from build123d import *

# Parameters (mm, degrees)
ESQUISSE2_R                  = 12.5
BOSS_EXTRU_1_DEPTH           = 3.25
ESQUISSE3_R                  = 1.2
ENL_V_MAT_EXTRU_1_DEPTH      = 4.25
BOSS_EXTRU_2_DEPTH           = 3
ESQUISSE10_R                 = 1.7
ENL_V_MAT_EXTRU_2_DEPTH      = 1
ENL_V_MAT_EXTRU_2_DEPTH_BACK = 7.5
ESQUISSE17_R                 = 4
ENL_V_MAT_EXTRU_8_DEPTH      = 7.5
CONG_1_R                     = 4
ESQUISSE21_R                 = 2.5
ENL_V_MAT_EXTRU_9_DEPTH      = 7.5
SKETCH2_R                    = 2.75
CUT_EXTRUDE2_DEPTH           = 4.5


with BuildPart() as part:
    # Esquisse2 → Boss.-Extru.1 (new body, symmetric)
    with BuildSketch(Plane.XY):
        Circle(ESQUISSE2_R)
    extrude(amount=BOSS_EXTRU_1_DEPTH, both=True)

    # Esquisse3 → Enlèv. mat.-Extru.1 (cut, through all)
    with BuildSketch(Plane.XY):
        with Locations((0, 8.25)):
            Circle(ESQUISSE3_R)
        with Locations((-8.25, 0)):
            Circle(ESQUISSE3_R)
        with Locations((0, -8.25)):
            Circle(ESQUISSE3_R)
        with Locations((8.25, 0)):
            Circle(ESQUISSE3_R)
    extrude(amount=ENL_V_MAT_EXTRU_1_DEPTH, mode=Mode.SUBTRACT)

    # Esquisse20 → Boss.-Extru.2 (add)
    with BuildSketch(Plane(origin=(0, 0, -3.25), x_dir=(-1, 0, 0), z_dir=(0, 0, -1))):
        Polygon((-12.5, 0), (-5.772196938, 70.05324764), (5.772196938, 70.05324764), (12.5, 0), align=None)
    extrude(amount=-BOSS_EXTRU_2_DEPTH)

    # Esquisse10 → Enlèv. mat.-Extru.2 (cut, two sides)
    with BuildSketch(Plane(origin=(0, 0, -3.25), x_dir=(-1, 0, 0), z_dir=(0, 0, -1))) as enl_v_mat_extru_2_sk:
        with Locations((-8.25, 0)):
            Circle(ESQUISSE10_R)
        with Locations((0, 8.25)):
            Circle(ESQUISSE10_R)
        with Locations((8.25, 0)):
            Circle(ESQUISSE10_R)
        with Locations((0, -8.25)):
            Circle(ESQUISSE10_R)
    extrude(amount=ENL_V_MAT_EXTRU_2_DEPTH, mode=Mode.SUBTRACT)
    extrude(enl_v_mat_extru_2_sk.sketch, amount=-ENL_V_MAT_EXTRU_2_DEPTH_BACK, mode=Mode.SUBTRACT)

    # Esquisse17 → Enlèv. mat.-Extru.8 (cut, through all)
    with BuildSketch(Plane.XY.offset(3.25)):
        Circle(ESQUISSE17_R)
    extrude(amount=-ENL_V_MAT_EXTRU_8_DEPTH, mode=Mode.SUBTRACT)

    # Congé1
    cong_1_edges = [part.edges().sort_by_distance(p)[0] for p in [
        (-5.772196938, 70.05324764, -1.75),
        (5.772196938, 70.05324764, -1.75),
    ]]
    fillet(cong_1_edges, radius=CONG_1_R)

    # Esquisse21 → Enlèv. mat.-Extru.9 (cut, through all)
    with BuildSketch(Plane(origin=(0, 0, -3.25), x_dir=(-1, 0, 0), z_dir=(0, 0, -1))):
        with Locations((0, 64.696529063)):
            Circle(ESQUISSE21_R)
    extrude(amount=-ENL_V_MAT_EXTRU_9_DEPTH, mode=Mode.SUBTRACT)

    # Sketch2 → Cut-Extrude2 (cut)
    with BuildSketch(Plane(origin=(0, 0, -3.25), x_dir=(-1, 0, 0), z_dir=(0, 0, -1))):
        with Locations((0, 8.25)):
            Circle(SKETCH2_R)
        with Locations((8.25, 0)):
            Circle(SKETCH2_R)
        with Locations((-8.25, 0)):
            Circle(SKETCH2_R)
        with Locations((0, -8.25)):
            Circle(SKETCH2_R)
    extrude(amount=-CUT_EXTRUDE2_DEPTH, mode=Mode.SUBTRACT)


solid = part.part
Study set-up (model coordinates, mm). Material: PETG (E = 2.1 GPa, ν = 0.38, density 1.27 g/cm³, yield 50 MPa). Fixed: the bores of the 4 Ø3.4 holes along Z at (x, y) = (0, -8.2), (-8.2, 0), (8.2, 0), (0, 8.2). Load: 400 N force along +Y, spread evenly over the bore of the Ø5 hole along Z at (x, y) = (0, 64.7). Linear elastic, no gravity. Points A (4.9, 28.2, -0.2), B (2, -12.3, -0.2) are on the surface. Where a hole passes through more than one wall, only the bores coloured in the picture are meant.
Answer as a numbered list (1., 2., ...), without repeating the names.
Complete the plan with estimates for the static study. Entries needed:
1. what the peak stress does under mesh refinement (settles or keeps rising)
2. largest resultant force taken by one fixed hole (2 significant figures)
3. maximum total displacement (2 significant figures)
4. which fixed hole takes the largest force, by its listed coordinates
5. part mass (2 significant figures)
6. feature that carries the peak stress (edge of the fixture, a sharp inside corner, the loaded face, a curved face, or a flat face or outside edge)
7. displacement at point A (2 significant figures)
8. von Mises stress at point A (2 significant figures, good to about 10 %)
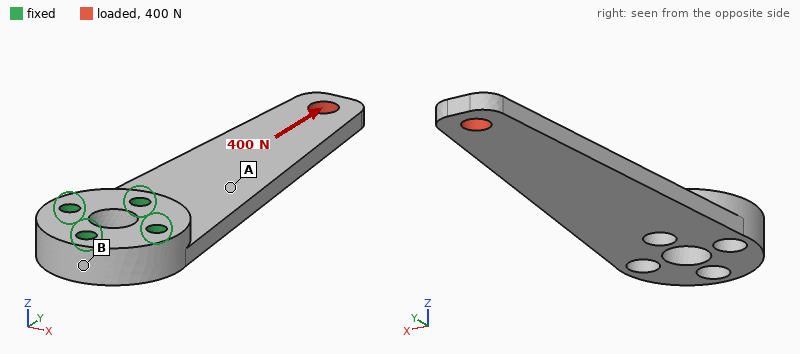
1. keeps rising
2. 150 N
3. 0.62 mm
4. (0, 8.2)
5. 6.8 g
6. edge of the fixture
7. 0.20 mm
8. 6.9 MPa
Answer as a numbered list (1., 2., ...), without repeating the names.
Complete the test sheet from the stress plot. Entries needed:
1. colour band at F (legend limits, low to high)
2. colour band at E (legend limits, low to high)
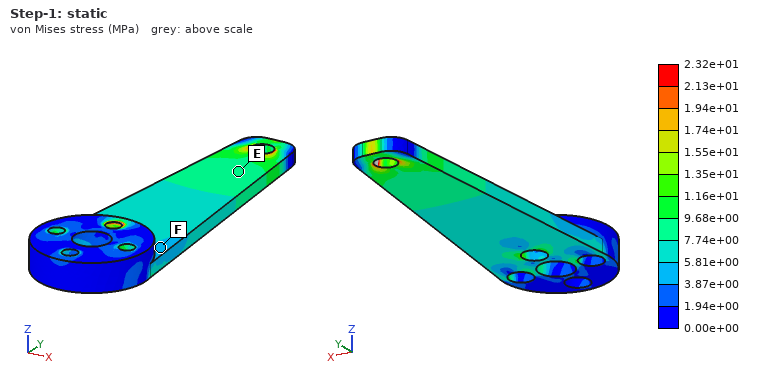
1. 3.87e+00 to 5.81e+00 MPa
2. 7.74e+00 to 9.68e+00 MPa
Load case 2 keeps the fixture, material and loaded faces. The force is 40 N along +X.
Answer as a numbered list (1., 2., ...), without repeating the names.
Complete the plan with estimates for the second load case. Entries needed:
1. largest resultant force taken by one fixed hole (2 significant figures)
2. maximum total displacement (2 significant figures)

1. 94 N
2. 0.94 mm
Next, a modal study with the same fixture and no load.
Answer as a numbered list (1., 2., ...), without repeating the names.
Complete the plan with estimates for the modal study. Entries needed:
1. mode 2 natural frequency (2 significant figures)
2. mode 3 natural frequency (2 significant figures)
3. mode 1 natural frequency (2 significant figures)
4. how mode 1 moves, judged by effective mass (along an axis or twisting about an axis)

1. 1100 Hz
2. 1200 Hz
3. 220 Hz
4. along Z
